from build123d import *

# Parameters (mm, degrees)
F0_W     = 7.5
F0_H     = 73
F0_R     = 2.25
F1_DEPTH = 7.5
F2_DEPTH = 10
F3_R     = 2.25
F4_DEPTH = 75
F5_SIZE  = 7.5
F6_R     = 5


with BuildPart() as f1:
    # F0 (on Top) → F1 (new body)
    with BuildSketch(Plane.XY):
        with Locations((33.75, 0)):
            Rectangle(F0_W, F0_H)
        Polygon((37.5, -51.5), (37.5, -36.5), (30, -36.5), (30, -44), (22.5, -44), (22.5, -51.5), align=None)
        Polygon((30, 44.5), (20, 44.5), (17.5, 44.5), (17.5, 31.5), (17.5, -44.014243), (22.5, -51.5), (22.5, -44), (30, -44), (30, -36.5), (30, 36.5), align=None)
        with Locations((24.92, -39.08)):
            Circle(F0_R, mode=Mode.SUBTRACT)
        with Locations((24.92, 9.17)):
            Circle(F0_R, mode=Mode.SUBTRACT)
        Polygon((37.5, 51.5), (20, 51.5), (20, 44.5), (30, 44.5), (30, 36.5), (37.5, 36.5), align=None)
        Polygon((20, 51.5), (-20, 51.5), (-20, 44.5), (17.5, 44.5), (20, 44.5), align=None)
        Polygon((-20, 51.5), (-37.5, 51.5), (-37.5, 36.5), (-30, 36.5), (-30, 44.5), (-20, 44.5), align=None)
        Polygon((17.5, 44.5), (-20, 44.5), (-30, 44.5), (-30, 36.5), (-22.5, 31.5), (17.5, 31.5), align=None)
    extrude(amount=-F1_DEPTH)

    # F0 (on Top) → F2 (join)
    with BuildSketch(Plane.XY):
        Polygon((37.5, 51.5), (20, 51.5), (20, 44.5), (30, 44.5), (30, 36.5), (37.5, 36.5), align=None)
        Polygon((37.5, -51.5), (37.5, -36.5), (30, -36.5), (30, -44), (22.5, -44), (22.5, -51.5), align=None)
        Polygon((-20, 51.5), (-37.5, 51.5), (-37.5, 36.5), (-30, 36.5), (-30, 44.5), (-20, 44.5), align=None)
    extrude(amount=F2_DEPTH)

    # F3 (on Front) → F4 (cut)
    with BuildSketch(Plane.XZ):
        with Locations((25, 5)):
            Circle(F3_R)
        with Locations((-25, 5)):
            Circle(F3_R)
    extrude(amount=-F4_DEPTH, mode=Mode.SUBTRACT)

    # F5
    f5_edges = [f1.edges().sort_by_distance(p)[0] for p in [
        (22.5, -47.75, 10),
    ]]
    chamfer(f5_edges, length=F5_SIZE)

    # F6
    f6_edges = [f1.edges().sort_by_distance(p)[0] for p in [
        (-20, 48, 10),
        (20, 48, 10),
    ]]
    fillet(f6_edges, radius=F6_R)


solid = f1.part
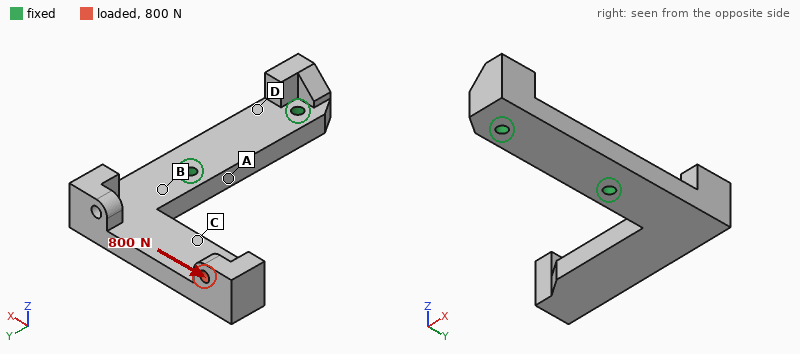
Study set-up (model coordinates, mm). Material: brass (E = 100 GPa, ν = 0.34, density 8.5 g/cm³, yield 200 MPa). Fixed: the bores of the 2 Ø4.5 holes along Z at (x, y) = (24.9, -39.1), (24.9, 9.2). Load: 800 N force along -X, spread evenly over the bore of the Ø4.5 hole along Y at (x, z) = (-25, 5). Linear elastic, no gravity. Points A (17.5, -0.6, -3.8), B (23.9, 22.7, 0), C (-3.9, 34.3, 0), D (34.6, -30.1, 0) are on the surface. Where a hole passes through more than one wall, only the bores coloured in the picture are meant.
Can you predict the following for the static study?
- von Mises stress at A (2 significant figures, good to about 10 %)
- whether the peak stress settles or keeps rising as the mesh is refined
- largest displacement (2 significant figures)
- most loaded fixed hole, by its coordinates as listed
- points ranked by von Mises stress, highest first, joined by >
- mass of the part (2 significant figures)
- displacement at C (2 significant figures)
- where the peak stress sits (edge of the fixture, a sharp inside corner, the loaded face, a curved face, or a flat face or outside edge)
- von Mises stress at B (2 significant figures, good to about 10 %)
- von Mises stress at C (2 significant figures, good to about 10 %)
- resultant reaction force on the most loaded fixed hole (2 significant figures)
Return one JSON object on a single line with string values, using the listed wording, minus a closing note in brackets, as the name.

{"von Mises stress at A": "21 MPa", "whether the peak stress settles or keeps rising as the mesh is refined": "keeps rising", "largest displacement": "0.39 mm", "most loaded fixed hole, by its coordinates as listed": "(24.9, 9.2)", "points ranked by von Mises stress, highest first, joined by >": "B > C > A > D", "mass of the part": "240 g", "displacement at C": "0.13 mm", "where the peak stress sits": "edge of the fixture", "von Mises stress at B": "53 MPa", "von Mises stress at C": "35 MPa", "resultant reaction force on the most loaded fixed hole": "1.3 kN"}
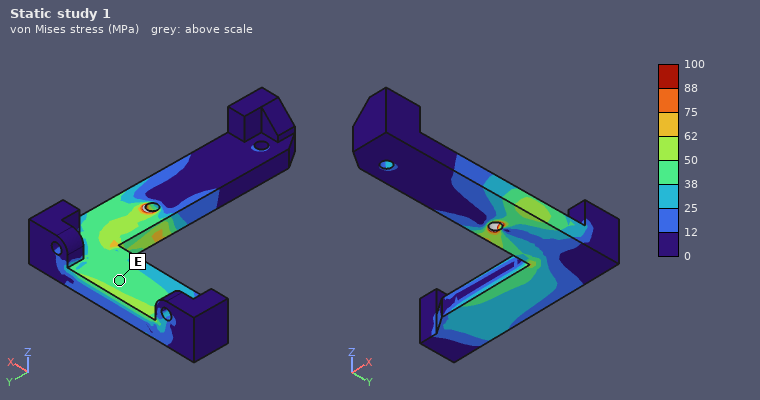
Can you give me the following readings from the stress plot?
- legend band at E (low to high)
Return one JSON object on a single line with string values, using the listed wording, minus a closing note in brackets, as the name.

{"legend band at E": "38 to 50 MPa"}
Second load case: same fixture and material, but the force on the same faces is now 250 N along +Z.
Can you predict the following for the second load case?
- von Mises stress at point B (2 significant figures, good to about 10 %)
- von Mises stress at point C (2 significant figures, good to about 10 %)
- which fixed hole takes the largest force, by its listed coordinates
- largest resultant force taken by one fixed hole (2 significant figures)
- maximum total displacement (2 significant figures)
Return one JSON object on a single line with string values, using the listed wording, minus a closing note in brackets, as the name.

{"von Mises stress at point B": "80 MPa", "von Mises stress at point C": "29 MPa", "which fixed hole takes the largest force, by its listed coordinates": "(24.9, 9.2)", "largest resultant force taken by one fixed hole": "260 N", "maximum total displacement": "0.56 mm"}
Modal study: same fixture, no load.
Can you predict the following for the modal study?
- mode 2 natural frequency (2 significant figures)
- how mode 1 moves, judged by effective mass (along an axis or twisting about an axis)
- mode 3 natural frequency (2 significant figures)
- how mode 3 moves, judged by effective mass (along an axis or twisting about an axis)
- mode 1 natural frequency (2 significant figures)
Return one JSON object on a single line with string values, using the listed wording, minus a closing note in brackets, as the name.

{"mode 2 natural frequency": "1100 Hz", "how mode 1 moves, judged by effective mass": "along Z", "mode 3 natural frequency": "1500 Hz", "how mode 3 moves, judged by effective mass": "along Z", "mode 1 natural frequency": "530 Hz"}
